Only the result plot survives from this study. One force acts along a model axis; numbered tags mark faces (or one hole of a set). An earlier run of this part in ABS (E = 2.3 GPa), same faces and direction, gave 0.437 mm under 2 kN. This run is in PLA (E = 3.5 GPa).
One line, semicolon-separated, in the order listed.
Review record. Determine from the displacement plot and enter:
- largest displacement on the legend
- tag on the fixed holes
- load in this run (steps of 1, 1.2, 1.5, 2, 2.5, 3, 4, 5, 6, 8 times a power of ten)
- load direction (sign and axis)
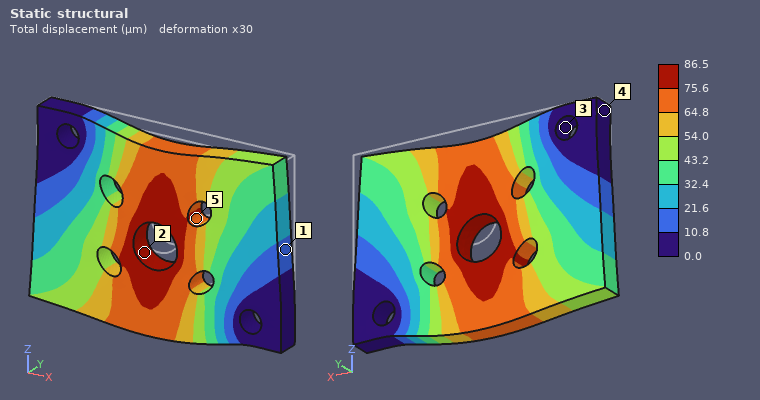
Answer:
86.5 µm; 3; 600 N; -Z
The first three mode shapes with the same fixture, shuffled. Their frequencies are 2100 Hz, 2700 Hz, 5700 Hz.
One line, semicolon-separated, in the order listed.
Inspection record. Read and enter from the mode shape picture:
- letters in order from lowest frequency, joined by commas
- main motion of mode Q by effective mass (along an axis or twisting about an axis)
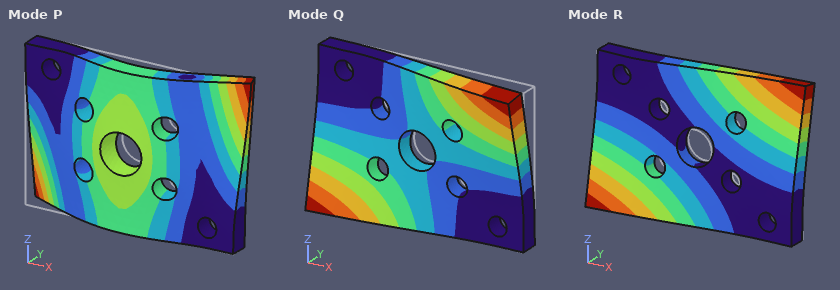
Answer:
R, Q, P; along Y
